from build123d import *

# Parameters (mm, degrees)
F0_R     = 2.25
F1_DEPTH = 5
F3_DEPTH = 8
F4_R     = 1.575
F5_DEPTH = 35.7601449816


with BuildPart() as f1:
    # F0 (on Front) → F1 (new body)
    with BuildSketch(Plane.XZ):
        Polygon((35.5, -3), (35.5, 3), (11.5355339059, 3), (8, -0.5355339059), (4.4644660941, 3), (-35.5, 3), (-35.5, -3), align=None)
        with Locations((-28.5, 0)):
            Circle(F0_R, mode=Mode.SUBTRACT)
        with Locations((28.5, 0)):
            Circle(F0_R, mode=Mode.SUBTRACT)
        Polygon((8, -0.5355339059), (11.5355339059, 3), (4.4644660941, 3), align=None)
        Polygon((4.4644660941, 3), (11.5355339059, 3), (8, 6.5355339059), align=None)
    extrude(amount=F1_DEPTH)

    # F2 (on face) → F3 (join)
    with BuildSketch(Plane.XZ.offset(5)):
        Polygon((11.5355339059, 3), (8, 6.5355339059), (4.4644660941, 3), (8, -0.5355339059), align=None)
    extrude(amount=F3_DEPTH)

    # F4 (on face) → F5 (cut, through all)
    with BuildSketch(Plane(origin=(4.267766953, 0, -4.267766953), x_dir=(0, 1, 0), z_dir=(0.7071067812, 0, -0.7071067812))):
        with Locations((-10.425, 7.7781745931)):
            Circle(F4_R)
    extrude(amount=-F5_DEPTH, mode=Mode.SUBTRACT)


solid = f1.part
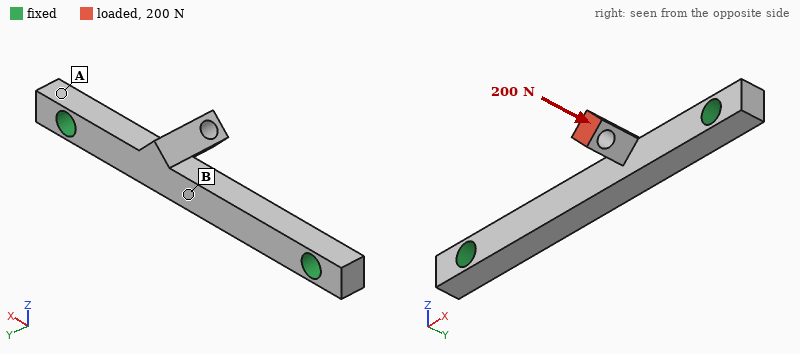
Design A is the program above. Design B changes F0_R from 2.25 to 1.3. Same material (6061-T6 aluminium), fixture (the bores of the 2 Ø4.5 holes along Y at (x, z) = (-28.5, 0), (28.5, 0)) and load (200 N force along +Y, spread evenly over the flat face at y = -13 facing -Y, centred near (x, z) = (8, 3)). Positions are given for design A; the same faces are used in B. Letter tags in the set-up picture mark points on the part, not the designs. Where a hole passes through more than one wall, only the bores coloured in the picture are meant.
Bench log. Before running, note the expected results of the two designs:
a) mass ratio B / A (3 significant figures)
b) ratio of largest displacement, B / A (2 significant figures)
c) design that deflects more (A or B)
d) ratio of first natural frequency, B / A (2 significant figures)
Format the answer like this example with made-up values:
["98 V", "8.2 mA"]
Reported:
["1.05", "1.1", "B", "0.92"]
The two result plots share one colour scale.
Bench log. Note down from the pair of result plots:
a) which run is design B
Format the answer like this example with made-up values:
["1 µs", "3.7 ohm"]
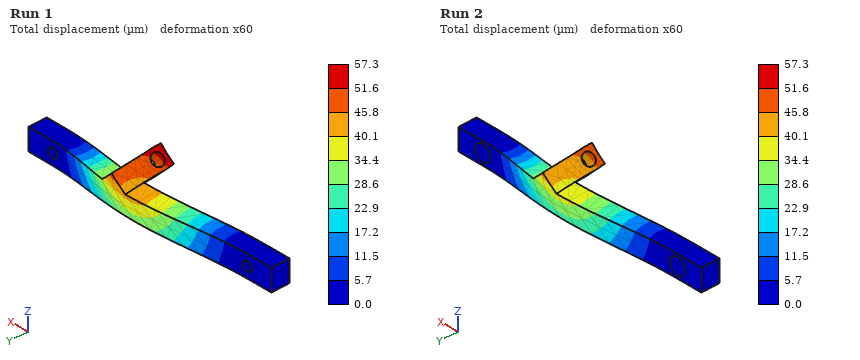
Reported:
["Run 1"]
